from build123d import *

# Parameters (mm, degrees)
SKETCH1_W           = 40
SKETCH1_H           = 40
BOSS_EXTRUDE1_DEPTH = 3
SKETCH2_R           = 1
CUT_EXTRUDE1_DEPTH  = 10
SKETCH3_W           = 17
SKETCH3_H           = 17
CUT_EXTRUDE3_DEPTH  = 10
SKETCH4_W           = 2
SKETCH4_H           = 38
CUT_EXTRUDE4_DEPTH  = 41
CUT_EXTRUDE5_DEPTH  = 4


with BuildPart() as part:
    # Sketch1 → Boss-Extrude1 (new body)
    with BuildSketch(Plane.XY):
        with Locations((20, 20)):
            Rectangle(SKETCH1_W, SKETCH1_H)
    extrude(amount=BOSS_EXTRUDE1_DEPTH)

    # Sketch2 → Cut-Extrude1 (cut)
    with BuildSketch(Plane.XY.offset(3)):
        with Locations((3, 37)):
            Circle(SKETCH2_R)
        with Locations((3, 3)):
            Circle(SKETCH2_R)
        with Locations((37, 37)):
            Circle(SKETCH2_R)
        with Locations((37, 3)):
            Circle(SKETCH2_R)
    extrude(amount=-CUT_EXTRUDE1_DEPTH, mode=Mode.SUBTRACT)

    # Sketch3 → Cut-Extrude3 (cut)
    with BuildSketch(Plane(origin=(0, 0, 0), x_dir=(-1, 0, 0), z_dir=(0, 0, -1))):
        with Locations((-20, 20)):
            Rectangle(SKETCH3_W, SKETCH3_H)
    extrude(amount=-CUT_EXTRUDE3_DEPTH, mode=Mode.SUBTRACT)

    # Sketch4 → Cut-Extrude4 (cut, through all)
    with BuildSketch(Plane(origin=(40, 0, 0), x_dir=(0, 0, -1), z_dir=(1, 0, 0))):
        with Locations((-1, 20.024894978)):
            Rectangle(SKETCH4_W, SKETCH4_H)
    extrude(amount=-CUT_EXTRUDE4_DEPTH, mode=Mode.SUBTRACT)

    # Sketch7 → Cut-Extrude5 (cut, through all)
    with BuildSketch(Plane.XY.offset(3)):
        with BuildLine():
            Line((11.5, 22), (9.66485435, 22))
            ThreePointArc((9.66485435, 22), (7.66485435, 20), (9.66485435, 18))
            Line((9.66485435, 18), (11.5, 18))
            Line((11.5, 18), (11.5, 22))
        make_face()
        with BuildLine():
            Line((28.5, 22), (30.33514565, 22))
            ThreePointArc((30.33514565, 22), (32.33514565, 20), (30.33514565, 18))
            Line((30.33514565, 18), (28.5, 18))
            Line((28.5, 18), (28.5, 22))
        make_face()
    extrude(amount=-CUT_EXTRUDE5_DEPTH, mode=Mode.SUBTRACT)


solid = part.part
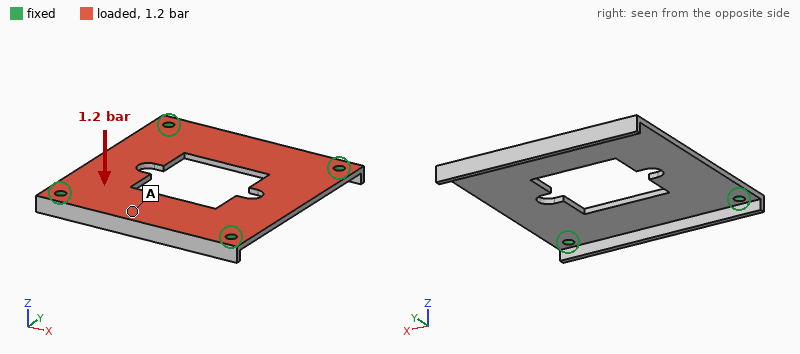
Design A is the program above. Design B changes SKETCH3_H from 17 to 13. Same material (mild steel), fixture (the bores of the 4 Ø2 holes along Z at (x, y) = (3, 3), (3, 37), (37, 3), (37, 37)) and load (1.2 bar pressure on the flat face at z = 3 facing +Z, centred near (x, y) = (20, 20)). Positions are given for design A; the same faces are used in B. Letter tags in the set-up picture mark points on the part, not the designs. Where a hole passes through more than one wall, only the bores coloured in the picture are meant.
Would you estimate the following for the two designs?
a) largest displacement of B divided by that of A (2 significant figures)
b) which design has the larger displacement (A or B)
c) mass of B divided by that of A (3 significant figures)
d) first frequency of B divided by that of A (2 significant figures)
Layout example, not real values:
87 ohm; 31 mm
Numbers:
1.1; B; 1.05; 0.93
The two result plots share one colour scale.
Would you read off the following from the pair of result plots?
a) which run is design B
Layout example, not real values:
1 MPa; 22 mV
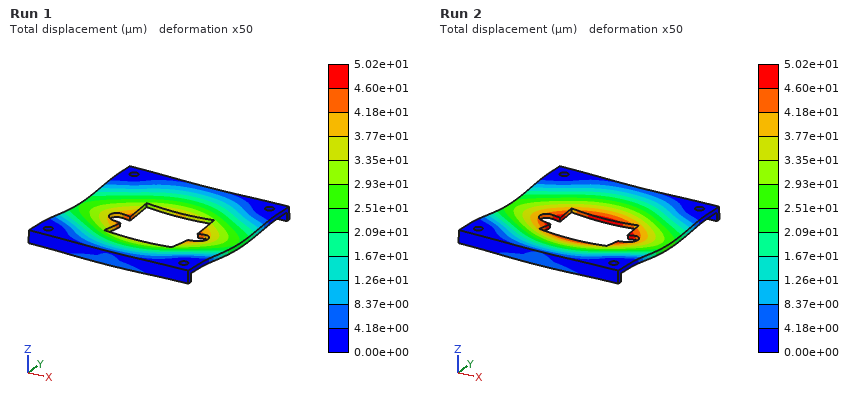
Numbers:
Run 2
